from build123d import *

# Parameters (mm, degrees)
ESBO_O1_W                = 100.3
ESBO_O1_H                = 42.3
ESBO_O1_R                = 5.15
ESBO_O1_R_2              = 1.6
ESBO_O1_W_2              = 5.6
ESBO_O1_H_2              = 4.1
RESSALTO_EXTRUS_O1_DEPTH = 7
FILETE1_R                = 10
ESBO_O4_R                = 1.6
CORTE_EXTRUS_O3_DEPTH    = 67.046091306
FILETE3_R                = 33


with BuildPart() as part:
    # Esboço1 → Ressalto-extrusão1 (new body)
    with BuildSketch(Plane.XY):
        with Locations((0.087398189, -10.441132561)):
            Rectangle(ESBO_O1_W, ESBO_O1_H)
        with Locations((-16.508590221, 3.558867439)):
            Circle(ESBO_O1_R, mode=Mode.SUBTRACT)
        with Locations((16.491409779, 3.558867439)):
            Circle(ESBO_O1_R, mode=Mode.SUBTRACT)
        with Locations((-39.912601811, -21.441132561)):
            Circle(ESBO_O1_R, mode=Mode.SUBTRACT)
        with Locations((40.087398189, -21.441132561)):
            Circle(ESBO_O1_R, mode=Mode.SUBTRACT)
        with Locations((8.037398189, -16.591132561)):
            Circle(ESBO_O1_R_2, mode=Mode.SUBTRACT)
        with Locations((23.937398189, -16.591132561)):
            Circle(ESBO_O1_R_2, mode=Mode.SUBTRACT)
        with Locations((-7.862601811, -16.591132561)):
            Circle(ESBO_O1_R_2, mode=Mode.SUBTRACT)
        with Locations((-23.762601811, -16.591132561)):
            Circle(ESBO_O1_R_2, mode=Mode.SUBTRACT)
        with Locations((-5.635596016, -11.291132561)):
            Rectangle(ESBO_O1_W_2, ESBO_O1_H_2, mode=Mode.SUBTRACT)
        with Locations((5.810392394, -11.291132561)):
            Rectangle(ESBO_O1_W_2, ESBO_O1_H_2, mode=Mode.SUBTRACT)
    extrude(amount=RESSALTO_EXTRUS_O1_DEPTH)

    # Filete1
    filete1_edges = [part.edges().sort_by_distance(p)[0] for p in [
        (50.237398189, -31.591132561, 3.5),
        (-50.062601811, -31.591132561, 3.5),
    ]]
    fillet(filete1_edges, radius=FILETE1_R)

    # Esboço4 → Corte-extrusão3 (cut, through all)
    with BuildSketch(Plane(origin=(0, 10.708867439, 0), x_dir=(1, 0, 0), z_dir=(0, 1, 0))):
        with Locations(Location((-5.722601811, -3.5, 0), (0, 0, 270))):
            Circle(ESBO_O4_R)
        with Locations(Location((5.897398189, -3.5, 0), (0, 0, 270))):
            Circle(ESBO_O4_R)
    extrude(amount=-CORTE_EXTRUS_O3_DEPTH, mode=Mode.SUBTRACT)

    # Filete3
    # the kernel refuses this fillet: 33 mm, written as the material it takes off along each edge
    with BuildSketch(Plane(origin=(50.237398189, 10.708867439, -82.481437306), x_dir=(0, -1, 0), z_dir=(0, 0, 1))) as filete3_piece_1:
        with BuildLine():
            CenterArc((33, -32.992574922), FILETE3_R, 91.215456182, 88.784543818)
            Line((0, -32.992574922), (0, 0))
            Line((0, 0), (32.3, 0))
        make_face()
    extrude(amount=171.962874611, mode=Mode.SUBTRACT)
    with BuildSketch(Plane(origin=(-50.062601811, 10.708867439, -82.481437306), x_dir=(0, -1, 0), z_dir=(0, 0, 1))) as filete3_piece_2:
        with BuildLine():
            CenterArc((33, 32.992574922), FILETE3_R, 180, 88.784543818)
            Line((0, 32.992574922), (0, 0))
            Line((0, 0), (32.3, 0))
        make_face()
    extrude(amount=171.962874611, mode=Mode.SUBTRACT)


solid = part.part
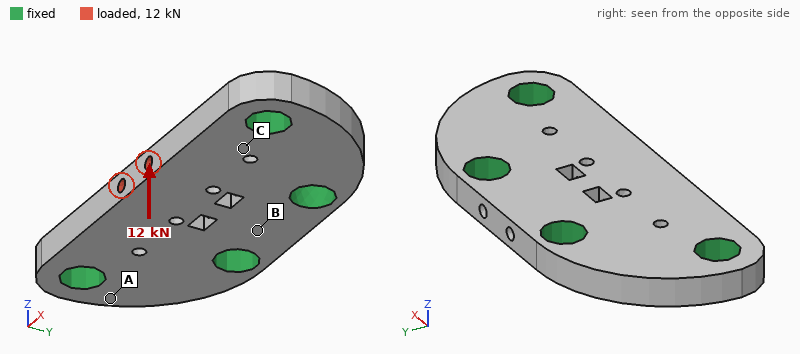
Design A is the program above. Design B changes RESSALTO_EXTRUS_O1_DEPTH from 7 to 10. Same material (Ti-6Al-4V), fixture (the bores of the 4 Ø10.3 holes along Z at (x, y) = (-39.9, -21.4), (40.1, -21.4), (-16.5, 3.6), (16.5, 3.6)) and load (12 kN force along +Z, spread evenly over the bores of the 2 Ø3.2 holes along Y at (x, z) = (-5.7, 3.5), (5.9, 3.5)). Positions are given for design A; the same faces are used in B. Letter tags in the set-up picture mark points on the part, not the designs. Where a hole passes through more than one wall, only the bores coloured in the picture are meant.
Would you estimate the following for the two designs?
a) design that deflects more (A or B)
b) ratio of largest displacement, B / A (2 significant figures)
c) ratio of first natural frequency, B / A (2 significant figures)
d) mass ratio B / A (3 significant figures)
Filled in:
A
0.40
1.3
1.44
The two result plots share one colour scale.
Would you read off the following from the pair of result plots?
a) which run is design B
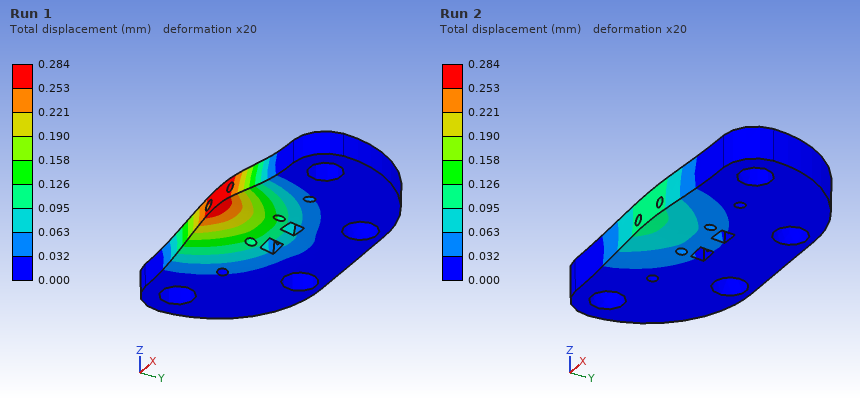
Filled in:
Run 2
